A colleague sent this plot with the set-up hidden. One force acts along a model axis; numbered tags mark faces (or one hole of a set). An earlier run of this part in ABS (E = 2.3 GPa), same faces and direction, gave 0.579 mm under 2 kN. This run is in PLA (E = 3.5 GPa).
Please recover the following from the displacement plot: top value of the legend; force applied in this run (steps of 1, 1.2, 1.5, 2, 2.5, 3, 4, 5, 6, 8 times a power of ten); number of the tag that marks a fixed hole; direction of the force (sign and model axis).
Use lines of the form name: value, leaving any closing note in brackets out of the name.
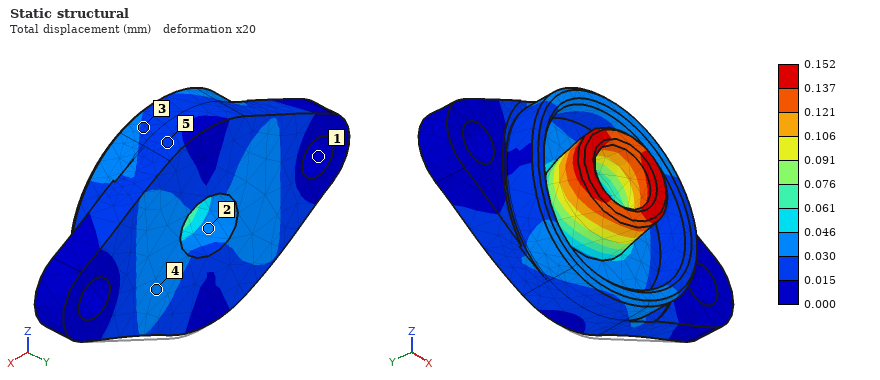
top value of the legend: 0.152 mm
force applied in this run: 800 N
number of the tag that marks a fixed hole: 1
direction of the force: -X
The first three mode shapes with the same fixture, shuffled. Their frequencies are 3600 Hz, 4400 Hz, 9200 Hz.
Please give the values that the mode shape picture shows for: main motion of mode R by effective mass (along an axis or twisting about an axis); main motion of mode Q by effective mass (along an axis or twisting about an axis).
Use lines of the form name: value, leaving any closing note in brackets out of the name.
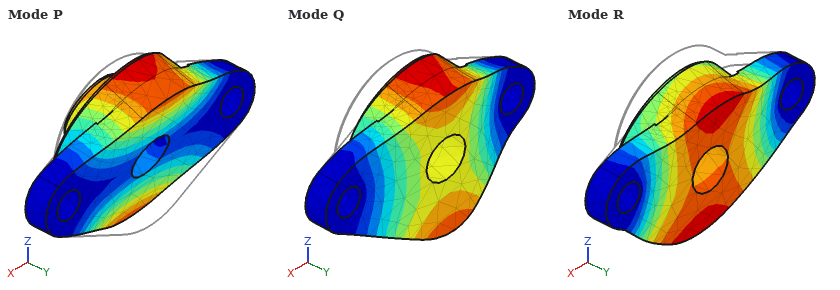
main motion of mode R by effective mass: along Z
main motion of mode Q by effective mass: along Y
